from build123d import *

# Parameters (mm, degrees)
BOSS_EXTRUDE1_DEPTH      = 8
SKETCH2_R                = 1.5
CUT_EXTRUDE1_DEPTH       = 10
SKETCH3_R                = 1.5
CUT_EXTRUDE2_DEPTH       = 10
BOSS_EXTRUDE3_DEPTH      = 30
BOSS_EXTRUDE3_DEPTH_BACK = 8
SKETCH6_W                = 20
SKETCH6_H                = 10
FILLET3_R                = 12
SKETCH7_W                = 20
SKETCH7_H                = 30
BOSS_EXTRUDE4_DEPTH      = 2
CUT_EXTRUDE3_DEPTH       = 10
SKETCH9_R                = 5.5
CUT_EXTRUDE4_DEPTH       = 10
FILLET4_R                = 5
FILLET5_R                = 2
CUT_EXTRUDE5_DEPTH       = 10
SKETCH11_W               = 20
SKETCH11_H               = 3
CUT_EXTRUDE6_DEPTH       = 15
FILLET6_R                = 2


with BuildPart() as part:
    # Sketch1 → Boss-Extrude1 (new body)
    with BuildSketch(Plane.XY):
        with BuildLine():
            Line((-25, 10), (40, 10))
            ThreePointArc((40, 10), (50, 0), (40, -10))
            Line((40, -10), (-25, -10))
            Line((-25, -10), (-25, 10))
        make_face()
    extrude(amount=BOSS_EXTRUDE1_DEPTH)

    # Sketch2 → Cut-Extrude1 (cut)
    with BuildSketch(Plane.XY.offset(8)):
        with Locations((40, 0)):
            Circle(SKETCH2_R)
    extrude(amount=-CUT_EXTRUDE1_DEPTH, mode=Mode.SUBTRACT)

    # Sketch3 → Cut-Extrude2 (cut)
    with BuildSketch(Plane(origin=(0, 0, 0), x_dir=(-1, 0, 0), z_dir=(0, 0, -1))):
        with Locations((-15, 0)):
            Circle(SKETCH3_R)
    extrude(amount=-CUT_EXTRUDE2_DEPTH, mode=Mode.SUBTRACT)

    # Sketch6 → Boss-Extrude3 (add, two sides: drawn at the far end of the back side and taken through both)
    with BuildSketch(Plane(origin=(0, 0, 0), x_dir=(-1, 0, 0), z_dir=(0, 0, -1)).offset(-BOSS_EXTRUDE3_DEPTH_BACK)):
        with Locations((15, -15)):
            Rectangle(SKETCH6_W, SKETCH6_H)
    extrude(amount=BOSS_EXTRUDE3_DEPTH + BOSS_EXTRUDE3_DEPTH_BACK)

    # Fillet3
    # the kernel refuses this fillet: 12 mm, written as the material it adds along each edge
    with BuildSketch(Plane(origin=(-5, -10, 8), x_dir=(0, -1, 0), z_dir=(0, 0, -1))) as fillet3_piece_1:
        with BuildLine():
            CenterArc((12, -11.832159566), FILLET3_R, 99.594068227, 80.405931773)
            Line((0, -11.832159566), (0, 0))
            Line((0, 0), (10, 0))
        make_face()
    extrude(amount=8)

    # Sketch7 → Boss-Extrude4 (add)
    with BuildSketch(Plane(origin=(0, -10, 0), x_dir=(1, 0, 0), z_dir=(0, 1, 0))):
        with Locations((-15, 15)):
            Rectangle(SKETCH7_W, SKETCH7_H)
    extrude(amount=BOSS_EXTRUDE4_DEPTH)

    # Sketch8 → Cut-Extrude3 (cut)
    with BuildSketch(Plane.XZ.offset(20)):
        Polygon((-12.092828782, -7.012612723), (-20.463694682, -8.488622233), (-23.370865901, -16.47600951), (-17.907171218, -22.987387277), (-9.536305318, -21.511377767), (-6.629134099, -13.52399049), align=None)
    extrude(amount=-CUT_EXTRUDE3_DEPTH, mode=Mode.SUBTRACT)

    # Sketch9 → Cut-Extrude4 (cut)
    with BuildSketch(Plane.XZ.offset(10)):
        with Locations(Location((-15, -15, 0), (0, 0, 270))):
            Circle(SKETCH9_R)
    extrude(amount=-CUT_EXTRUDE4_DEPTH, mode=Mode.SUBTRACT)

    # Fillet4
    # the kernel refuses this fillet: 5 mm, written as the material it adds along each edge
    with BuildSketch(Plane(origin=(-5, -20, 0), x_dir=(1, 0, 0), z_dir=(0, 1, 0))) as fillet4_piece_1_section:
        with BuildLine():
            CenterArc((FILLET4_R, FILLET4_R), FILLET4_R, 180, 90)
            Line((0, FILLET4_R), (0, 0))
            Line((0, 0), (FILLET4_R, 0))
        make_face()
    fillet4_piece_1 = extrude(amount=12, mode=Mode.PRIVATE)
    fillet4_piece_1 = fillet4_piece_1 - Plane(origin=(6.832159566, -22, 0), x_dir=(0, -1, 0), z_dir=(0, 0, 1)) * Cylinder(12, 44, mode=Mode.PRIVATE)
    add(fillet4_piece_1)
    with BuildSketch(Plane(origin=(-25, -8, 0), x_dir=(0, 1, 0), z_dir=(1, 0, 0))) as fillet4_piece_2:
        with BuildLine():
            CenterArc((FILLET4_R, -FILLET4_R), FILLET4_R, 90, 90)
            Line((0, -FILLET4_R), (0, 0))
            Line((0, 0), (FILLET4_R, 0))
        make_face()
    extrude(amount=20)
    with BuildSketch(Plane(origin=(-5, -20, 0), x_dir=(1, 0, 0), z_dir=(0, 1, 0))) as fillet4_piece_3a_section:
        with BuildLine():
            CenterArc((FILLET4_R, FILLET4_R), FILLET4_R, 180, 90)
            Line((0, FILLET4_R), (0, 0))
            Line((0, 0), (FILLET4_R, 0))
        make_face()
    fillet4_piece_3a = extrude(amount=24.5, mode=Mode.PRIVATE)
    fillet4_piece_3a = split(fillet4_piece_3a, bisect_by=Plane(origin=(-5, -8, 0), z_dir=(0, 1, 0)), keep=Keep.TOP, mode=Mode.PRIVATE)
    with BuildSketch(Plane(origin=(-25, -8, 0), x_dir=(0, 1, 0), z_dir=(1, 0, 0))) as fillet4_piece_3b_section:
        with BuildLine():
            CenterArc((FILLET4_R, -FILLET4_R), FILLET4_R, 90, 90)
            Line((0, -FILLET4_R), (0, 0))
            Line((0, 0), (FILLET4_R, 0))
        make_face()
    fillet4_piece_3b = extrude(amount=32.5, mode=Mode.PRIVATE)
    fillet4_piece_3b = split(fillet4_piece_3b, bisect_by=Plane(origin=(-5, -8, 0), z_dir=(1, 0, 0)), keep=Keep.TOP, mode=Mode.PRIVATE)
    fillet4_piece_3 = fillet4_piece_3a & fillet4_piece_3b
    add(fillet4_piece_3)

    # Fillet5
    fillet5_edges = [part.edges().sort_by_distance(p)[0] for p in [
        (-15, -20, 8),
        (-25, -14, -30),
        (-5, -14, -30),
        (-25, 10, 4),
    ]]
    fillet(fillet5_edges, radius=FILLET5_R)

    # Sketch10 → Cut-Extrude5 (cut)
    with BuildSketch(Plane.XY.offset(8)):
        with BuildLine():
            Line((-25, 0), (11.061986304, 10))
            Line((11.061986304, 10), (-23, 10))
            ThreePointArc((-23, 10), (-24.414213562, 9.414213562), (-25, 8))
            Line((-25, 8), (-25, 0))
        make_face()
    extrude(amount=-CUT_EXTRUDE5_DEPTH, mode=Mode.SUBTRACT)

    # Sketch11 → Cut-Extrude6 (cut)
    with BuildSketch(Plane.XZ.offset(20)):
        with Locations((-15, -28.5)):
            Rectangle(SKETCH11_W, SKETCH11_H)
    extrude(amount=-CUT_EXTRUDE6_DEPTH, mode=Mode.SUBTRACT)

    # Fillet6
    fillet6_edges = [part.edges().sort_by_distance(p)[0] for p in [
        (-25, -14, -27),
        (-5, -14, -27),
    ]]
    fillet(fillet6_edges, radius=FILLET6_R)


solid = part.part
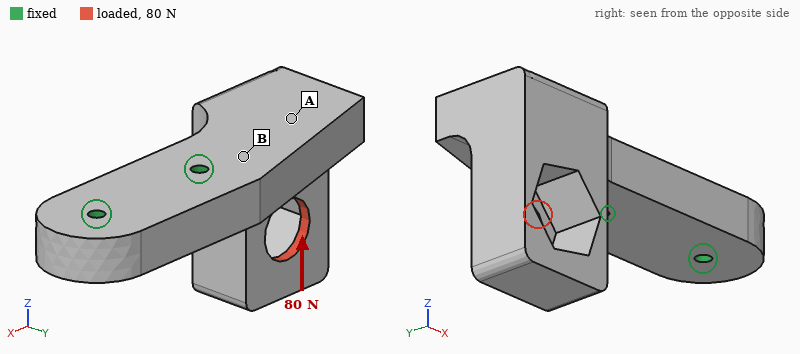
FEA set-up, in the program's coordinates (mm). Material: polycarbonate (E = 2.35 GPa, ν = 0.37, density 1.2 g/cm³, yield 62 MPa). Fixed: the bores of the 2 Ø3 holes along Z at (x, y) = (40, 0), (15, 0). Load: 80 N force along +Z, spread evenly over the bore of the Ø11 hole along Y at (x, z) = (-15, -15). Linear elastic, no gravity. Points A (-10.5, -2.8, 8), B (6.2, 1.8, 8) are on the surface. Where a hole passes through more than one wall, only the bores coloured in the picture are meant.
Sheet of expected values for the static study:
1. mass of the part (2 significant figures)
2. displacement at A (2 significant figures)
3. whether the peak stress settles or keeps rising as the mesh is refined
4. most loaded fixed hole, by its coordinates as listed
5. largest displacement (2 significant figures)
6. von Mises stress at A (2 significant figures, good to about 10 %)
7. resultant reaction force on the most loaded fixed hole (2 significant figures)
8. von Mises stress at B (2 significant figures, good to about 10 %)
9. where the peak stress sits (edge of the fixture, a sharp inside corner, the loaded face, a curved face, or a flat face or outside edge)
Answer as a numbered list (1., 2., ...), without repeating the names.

1. 20 g
2. 0.38 mm
3. keeps rising
4. (15, 0)
5. 1.0 mm
6. 2.1 MPa
7. 110 N
8. 8.6 MPa
9. edge of the fixture
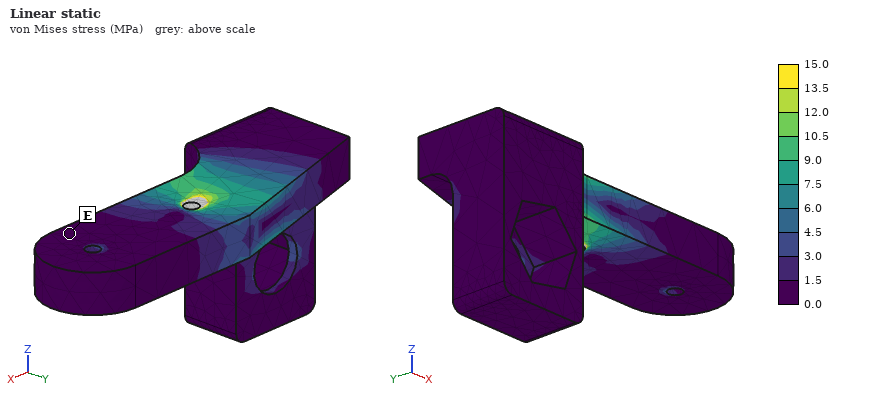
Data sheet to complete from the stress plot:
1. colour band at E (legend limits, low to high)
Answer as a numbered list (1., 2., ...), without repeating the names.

1. 0.0 to 1.5 MPa
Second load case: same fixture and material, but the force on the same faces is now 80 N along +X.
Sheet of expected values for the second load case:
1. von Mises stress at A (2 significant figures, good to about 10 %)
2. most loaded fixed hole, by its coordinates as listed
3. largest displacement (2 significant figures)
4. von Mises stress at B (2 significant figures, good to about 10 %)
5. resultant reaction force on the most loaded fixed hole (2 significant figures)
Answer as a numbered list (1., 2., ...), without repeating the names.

1. 3.3 MPa
2. (15, 0)
3. 0.94 mm
4. 7.1 MPa
5. 74 N
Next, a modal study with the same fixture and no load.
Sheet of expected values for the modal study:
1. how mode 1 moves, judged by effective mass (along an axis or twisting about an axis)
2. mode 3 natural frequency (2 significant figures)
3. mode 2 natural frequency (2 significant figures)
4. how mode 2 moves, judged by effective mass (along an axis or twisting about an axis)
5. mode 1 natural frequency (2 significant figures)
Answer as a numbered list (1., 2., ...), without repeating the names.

1. along Z
2. 1500 Hz
3. 760 Hz
4. along Y
5. 510 Hz
